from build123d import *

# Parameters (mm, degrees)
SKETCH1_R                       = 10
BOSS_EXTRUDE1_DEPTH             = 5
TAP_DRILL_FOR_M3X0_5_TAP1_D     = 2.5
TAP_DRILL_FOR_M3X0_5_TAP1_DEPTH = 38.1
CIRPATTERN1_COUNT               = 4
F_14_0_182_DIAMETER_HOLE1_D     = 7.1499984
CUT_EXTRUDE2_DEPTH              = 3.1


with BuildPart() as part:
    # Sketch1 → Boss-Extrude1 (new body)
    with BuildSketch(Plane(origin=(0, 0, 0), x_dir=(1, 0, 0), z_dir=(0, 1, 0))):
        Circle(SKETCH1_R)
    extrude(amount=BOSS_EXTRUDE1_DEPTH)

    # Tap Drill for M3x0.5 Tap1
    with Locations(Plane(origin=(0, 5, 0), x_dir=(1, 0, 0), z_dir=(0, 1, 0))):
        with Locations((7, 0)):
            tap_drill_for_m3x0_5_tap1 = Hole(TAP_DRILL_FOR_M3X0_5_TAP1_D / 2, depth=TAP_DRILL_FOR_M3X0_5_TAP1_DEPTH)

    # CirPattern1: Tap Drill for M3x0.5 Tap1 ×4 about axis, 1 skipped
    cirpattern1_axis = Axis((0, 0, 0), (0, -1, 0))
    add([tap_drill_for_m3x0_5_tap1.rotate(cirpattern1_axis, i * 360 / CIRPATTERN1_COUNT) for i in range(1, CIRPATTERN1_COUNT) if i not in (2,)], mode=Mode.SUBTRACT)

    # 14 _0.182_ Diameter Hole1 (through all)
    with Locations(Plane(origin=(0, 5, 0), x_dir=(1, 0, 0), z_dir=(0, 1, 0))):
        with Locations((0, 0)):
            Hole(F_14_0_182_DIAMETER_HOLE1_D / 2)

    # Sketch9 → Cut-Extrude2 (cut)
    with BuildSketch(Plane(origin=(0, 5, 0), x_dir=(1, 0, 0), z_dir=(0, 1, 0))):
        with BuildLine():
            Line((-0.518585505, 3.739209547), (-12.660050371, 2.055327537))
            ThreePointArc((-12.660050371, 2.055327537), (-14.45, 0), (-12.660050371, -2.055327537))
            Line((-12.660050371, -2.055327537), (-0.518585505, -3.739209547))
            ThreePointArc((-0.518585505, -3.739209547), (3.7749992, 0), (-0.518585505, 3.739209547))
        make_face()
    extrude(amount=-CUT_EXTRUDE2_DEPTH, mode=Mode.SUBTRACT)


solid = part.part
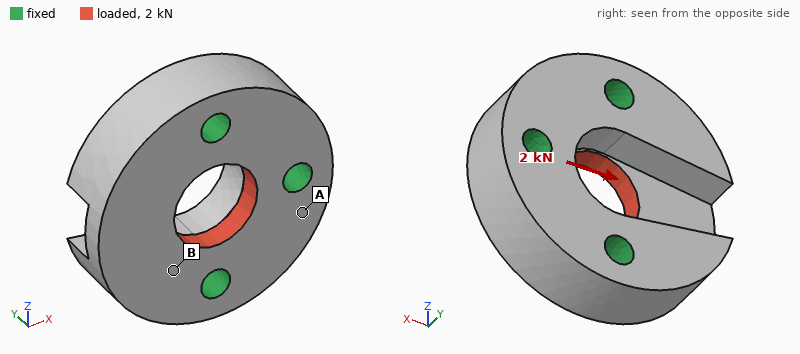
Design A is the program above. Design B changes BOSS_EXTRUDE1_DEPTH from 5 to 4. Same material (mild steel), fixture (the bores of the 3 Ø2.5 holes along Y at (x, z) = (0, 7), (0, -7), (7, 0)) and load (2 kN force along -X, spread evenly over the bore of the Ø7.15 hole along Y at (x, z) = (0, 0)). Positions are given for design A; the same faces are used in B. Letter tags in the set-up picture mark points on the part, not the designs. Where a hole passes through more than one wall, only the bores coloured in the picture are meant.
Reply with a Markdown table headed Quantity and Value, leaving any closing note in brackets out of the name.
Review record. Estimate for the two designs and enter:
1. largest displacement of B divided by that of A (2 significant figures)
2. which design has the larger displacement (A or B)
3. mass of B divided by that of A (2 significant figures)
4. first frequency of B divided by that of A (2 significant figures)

| Quantity | Value |
|---|---|
| largest displacement of B divided by that of A | 1.2 |
| which design has the larger displacement | B |
| mass of B divided by that of A | 0.81 |
| first frequency of B divided by that of A | 0.84 |
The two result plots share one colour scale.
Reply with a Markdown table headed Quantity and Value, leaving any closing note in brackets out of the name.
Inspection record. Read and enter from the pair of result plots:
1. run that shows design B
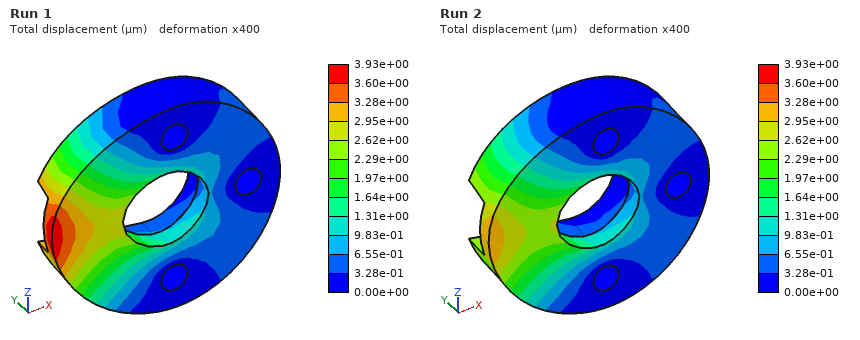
| Quantity | Value |
|---|---|
| run that shows design B | Run 1 |
